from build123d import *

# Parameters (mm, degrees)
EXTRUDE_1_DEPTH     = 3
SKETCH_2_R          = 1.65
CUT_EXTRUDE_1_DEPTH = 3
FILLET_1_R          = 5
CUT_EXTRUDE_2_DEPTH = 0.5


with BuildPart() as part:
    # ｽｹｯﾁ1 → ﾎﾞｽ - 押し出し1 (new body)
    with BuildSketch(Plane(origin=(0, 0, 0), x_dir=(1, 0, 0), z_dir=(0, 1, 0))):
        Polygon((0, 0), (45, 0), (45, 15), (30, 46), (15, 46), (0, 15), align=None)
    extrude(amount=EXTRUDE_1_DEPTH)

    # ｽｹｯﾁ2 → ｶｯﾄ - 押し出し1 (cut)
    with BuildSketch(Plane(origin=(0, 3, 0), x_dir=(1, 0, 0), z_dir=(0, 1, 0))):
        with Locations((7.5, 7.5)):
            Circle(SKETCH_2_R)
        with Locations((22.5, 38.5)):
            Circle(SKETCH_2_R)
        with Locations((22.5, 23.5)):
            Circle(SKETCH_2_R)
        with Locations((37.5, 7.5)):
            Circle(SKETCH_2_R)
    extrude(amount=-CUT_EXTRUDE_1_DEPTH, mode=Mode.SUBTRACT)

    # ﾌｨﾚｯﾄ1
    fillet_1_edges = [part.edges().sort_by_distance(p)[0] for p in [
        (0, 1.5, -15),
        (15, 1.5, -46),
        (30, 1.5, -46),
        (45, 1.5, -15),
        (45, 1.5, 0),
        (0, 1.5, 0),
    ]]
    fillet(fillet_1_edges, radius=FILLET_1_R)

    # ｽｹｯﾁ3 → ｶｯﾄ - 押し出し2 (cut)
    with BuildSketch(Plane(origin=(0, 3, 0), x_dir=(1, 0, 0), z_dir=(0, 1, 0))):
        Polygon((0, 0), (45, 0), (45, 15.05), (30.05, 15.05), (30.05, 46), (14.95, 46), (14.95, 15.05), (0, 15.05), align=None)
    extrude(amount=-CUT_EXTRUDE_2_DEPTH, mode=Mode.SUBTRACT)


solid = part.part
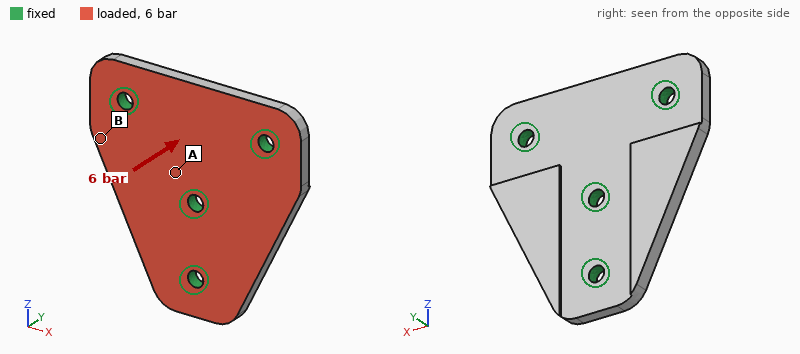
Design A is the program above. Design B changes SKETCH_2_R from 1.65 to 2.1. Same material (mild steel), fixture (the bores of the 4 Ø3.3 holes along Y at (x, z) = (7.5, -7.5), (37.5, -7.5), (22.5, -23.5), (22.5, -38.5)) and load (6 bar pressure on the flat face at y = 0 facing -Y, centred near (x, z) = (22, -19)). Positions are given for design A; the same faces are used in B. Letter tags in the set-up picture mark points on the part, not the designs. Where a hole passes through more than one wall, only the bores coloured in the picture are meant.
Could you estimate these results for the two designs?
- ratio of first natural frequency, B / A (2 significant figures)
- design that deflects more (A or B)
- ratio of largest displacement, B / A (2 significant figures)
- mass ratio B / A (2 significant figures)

1.1
A
0.90
0.99
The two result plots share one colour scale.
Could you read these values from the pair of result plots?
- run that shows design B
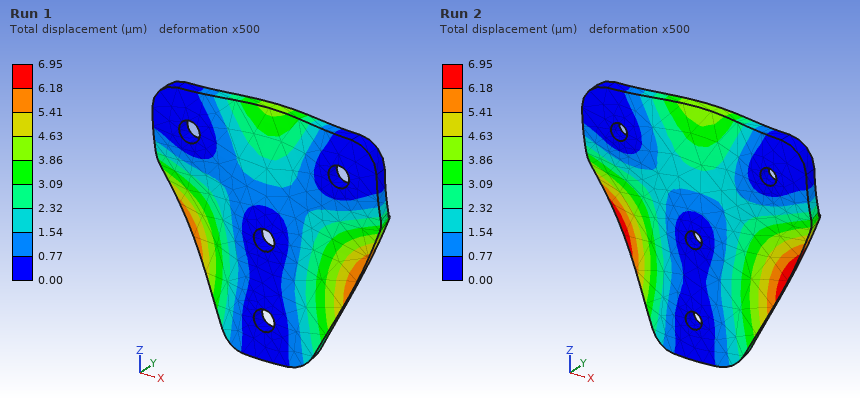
Run 1
